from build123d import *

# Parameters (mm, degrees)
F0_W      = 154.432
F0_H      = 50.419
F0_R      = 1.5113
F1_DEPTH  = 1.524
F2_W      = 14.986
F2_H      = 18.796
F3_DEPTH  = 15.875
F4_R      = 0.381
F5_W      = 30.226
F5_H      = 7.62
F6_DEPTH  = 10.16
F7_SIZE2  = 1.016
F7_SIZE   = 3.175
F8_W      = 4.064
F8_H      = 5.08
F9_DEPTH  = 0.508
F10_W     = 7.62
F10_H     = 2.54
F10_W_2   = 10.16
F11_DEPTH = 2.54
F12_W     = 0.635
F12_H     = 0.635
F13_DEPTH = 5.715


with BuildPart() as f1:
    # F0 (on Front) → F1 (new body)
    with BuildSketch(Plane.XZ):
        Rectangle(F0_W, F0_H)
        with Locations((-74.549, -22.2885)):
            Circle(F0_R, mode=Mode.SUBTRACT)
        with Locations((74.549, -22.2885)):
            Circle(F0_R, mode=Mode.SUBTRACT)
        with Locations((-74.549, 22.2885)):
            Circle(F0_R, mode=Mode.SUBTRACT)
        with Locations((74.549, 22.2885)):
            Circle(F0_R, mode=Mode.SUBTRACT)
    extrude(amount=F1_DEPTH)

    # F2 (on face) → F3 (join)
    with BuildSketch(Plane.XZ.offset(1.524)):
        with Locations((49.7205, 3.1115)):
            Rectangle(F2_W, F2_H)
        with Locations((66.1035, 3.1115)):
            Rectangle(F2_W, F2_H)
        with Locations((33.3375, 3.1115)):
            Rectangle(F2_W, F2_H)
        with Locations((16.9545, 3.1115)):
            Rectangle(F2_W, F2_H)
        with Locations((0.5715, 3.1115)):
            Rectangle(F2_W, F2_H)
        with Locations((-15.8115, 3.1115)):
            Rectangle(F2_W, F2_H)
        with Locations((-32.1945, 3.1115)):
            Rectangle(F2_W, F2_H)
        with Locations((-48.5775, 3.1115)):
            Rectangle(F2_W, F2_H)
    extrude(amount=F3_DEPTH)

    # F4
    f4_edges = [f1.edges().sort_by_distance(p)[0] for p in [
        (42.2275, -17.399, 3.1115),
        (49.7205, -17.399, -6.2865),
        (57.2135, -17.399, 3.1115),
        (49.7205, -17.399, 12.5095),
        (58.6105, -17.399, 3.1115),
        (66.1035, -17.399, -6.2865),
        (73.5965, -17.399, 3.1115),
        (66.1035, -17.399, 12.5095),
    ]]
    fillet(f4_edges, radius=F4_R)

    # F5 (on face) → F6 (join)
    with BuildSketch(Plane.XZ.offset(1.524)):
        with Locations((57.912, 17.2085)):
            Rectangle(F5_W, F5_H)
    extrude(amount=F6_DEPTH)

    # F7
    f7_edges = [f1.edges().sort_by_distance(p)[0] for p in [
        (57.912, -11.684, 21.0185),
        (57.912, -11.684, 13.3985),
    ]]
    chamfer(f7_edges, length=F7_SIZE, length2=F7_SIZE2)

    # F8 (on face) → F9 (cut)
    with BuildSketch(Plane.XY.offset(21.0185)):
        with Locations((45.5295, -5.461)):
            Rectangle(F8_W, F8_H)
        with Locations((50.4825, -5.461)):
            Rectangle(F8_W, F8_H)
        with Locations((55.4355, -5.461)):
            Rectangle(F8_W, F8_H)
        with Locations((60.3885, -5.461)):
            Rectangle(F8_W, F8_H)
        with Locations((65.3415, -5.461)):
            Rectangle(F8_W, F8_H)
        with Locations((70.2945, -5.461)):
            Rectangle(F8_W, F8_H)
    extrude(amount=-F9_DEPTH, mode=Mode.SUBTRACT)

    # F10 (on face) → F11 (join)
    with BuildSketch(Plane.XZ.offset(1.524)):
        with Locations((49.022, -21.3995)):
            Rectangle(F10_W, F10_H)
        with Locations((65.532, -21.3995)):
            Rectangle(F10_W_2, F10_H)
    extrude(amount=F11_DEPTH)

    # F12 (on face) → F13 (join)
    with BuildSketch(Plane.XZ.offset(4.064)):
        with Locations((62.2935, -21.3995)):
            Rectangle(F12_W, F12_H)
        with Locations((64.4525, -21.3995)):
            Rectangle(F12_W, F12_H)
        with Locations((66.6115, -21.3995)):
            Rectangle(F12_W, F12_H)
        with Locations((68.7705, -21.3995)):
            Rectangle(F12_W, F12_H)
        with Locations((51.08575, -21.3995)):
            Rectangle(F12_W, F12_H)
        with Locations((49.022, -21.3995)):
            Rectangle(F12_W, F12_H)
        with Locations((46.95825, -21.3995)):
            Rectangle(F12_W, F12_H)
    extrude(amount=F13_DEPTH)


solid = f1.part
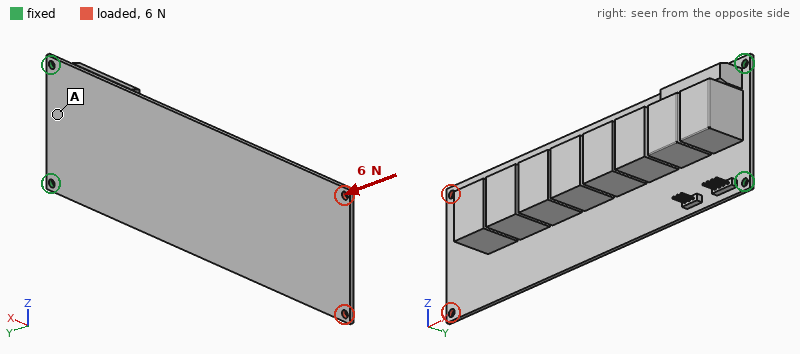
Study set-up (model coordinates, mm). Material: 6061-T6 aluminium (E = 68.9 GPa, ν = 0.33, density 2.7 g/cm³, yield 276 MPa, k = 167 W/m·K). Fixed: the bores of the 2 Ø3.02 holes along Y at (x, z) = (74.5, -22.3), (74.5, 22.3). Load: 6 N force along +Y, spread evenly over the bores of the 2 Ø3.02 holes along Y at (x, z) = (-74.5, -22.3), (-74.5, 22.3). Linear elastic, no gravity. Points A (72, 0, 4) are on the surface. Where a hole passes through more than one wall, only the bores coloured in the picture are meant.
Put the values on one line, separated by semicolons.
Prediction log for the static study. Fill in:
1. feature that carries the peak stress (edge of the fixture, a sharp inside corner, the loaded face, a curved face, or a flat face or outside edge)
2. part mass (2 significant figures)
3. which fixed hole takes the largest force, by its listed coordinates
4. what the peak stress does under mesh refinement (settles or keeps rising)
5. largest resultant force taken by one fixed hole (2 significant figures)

edge of the fixture; 130 g; (74.5, -22.3); keeps rising; 8.1 N
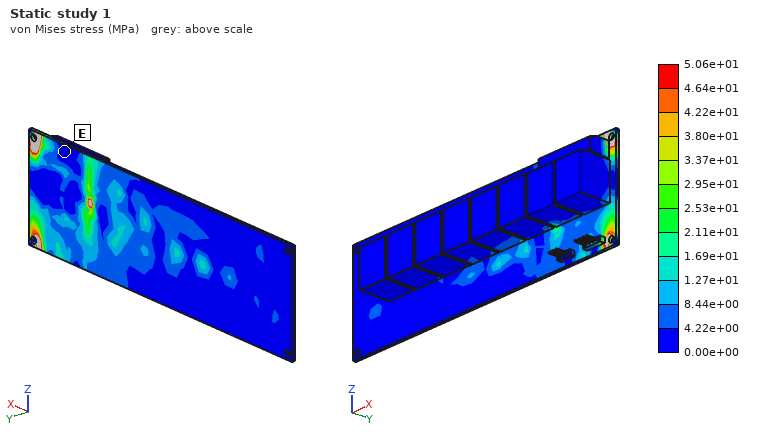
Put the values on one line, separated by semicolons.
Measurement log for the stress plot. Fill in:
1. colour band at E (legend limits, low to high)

0.00e+00 to 4.22e+00 MPa
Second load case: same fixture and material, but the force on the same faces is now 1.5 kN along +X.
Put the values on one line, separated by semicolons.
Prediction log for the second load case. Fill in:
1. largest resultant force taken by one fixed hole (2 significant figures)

790 N
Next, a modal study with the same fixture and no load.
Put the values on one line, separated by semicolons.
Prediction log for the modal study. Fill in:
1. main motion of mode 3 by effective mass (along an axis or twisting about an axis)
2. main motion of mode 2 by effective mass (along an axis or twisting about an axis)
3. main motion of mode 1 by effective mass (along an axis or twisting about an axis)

along Z; along Y; along Y
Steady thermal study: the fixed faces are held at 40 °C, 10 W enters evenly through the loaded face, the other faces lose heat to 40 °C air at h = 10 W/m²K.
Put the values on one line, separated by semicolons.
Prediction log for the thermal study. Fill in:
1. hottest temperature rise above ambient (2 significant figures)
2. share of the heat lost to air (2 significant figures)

69 K; 54 %
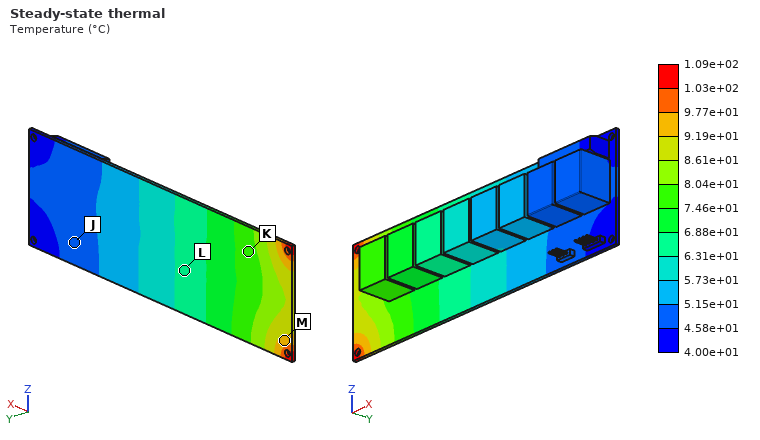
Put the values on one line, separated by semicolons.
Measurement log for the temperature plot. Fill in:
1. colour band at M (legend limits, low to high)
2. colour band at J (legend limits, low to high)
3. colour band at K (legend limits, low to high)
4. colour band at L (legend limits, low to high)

9.19e+01 to 9.77e+01 °C; 4.58e+01 to 5.15e+01 °C; 7.46e+01 to 8.04e+01 °C; 6.31e+01 to 6.88e+01 °C
